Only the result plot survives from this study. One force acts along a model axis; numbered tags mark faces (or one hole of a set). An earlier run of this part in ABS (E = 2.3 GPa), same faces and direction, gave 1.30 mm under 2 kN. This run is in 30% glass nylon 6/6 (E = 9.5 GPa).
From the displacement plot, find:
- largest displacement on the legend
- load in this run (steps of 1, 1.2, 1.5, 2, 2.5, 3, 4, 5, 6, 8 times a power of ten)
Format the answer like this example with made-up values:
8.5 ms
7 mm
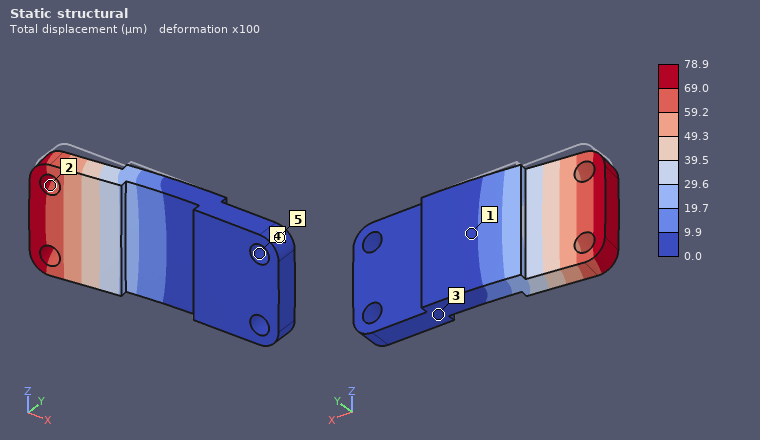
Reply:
78.9 µm
500 N
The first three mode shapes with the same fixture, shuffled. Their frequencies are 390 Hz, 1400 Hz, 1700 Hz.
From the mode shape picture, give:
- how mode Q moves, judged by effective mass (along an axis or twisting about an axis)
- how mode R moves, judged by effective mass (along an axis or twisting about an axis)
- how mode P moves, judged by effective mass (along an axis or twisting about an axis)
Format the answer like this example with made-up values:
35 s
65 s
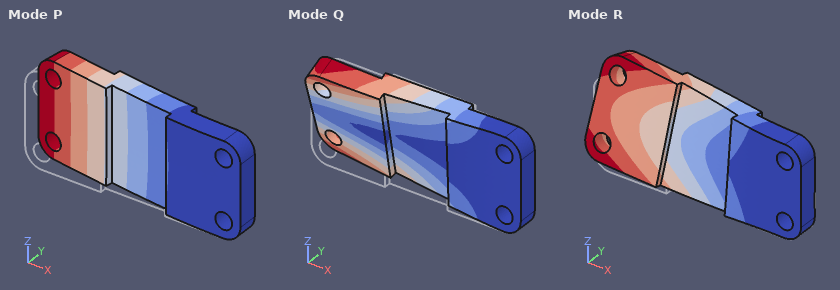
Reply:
along Z
along Z
along Y
